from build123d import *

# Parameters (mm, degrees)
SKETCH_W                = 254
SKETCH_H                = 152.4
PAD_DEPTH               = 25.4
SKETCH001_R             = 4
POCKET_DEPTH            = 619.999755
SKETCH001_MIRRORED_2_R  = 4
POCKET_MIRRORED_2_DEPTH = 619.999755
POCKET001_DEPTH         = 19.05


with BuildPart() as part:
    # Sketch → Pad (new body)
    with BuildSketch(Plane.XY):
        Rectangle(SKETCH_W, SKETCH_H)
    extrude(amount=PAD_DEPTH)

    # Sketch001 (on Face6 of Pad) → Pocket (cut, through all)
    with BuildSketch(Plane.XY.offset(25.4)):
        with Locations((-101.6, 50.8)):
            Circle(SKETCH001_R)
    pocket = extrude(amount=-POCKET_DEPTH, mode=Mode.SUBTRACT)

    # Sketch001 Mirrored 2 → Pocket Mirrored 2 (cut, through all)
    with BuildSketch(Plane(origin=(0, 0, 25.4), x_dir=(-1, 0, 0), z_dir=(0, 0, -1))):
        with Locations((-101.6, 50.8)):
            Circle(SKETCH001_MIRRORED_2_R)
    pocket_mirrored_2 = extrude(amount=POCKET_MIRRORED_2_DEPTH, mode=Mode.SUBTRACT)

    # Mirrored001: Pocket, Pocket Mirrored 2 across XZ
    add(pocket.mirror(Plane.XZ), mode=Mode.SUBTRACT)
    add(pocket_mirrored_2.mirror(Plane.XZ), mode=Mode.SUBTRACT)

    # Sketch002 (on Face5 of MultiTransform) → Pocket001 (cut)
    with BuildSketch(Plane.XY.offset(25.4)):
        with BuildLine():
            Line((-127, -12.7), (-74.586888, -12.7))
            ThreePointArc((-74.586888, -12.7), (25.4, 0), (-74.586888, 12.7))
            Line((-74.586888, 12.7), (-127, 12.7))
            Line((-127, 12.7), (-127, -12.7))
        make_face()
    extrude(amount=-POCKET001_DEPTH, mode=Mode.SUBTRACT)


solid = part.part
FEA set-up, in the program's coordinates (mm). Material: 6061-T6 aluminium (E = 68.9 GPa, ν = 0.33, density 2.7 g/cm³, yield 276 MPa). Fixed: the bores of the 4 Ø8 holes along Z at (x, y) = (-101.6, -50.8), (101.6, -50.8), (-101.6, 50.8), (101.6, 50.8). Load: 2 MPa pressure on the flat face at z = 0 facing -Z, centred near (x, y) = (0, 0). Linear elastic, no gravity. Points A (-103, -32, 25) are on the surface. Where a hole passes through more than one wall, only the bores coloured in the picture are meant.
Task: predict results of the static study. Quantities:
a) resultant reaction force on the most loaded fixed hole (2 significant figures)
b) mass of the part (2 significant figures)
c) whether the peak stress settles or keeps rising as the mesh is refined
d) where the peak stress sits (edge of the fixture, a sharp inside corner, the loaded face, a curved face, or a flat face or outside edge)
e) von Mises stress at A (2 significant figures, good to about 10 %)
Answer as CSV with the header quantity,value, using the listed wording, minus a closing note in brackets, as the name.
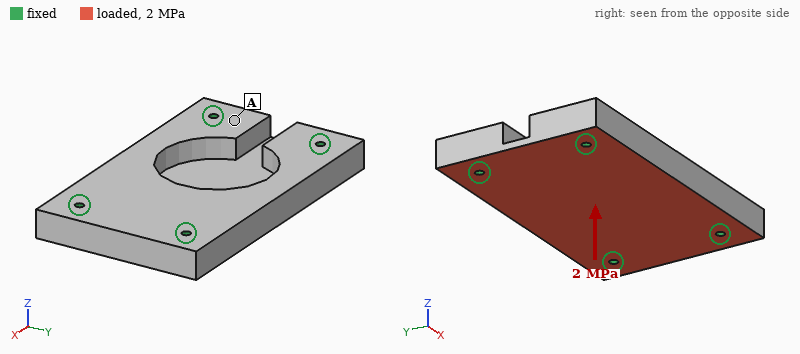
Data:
quantity,value
resultant reaction force on the most loaded fixed hole,21 kN
mass of the part,2.2 kg
whether the peak stress settles or keeps rising as the mesh is refined,keeps rising
where the peak stress sits,edge of the fixture
von Mises stress at A,25 MPa
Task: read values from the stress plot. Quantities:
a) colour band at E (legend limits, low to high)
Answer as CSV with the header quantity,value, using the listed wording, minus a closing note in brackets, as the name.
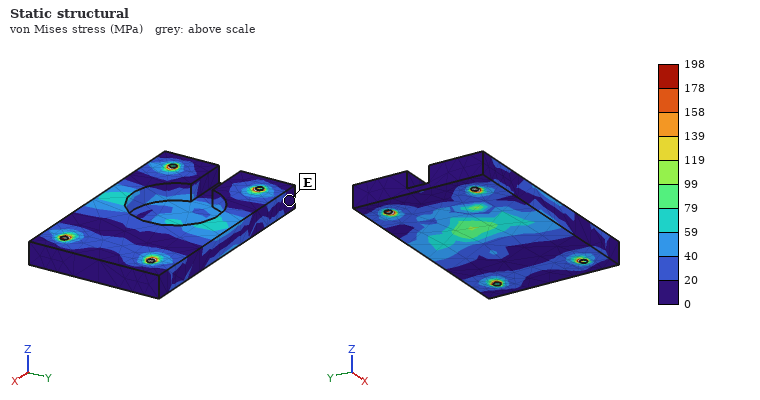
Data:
quantity,value
colour band at E,0 to 20 MPa
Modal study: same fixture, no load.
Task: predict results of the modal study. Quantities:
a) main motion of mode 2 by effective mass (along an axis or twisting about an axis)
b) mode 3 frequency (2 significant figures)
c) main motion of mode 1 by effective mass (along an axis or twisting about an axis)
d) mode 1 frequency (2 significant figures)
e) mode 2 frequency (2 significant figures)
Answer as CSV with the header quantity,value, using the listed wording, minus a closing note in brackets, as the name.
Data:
quantity,value
main motion of mode 2 by effective mass,twisting about X
mode 3 frequency,5100 Hz
main motion of mode 1 by effective mass,along Z
mode 1 frequency,2500 Hz
mode 2 frequency,3300 Hz
